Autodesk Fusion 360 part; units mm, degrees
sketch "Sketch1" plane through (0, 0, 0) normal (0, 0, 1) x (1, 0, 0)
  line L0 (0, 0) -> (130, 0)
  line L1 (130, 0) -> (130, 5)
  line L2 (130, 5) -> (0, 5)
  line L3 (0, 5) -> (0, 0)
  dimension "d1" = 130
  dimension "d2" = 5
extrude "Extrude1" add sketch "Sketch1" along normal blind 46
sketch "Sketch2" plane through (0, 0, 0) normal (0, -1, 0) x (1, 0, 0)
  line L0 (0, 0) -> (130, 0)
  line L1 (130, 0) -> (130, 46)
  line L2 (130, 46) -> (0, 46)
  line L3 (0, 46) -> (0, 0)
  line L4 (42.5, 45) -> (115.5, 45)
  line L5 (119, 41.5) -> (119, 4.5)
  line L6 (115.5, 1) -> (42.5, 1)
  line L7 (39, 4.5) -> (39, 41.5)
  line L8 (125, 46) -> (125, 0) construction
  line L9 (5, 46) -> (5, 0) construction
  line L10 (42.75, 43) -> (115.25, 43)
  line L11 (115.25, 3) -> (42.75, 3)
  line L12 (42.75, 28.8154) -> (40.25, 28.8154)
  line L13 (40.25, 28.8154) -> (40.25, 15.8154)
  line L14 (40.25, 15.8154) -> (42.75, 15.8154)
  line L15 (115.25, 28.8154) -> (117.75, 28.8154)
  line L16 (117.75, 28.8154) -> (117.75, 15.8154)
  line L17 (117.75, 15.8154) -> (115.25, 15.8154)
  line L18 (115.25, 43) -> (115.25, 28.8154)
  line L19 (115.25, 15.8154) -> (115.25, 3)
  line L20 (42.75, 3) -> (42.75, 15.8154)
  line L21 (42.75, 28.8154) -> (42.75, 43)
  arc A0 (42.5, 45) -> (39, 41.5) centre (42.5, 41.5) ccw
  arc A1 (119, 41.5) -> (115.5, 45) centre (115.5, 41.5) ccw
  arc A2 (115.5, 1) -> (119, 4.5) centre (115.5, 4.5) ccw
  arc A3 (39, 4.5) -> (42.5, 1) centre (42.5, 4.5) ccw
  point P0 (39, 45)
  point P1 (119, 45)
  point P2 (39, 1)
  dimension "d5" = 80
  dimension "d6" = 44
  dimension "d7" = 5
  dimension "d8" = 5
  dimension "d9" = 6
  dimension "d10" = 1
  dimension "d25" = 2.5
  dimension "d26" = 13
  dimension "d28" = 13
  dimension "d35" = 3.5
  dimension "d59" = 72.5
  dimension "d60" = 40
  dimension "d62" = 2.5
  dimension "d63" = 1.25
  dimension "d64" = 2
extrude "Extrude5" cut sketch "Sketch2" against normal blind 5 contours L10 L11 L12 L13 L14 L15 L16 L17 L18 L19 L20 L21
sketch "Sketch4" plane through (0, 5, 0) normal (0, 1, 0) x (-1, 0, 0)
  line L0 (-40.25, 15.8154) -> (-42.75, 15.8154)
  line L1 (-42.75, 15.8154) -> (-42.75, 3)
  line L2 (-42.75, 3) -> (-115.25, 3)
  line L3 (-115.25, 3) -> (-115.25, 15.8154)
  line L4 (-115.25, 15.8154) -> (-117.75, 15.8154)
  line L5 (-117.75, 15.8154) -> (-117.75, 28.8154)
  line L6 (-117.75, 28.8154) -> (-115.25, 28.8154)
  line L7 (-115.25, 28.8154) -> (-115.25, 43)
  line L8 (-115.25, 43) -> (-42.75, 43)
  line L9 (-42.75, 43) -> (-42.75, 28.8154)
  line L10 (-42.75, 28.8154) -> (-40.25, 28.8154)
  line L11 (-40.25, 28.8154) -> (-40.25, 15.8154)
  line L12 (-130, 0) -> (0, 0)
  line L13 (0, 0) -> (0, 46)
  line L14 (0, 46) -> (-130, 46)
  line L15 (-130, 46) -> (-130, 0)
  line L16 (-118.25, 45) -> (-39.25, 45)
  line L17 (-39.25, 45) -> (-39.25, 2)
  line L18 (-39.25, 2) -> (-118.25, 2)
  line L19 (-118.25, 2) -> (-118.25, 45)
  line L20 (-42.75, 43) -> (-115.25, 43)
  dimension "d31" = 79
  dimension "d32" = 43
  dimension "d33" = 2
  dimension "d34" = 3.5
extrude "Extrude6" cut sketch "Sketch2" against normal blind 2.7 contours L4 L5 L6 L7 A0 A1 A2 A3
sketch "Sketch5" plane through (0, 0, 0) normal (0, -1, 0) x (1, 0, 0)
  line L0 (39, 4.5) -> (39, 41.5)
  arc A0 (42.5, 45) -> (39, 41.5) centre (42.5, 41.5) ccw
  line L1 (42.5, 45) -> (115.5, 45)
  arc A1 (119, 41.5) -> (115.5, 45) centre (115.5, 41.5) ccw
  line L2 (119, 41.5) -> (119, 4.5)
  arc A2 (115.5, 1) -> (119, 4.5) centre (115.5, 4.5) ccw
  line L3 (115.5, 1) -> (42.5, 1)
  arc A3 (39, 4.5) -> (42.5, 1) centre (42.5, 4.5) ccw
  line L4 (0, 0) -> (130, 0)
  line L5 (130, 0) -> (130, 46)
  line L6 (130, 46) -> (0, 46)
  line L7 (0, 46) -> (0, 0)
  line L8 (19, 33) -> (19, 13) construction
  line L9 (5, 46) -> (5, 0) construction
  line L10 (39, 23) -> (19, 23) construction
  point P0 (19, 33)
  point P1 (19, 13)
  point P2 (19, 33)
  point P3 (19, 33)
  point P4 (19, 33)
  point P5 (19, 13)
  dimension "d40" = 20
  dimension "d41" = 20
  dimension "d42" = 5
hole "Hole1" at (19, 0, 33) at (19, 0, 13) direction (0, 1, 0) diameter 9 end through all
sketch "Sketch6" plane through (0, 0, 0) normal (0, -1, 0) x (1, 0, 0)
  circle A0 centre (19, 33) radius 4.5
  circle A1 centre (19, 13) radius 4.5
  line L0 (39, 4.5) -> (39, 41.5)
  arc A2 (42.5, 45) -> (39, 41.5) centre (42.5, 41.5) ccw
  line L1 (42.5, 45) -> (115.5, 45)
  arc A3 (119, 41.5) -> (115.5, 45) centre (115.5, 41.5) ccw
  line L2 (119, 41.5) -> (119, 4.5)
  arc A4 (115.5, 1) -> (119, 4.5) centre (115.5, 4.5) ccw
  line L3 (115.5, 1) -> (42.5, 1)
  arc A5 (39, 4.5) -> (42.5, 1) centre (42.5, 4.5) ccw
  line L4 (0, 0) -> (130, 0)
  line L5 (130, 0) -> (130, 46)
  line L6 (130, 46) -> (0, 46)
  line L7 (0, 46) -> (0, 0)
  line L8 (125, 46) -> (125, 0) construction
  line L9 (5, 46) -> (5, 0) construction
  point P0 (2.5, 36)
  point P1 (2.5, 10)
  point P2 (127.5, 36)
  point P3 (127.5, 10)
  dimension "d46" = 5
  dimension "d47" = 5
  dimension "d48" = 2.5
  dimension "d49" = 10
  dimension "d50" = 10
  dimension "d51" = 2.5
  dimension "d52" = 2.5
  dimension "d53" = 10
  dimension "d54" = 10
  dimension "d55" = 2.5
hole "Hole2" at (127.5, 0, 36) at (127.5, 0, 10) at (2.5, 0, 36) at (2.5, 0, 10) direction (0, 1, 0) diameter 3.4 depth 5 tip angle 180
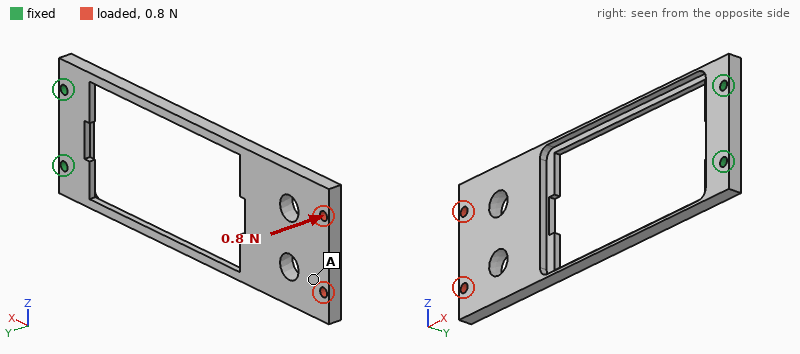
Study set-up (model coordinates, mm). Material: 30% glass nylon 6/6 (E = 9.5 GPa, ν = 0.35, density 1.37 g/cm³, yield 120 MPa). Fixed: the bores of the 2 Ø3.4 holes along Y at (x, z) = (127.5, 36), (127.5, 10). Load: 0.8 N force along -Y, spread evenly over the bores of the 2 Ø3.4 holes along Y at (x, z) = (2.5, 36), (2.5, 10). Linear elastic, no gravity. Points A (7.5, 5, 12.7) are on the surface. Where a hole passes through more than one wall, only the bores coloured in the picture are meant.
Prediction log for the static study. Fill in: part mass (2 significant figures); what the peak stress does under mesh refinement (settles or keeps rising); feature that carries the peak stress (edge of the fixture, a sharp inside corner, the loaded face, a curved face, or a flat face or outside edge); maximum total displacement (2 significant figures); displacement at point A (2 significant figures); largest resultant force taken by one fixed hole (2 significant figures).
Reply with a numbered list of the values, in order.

1. 18 g
2. keeps rising
3. a sharp inside corner
4. 1.4 mm
5. 1.3 mm
6. 1.3 N
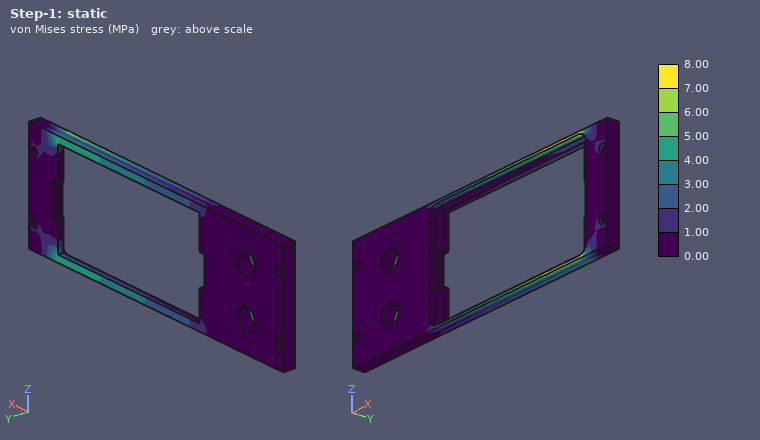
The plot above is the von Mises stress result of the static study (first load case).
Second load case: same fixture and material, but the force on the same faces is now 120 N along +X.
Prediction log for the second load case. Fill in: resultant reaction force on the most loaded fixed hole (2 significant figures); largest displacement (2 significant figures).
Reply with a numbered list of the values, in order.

1. 75 N
2. 1.6 mm
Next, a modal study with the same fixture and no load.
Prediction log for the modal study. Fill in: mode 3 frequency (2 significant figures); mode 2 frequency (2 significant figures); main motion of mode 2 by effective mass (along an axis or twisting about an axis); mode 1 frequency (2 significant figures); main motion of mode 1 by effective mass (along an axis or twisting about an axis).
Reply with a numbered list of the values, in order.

1. 200 Hz
2. 78 Hz
3. along Z
4. 44 Hz
5. along Y
